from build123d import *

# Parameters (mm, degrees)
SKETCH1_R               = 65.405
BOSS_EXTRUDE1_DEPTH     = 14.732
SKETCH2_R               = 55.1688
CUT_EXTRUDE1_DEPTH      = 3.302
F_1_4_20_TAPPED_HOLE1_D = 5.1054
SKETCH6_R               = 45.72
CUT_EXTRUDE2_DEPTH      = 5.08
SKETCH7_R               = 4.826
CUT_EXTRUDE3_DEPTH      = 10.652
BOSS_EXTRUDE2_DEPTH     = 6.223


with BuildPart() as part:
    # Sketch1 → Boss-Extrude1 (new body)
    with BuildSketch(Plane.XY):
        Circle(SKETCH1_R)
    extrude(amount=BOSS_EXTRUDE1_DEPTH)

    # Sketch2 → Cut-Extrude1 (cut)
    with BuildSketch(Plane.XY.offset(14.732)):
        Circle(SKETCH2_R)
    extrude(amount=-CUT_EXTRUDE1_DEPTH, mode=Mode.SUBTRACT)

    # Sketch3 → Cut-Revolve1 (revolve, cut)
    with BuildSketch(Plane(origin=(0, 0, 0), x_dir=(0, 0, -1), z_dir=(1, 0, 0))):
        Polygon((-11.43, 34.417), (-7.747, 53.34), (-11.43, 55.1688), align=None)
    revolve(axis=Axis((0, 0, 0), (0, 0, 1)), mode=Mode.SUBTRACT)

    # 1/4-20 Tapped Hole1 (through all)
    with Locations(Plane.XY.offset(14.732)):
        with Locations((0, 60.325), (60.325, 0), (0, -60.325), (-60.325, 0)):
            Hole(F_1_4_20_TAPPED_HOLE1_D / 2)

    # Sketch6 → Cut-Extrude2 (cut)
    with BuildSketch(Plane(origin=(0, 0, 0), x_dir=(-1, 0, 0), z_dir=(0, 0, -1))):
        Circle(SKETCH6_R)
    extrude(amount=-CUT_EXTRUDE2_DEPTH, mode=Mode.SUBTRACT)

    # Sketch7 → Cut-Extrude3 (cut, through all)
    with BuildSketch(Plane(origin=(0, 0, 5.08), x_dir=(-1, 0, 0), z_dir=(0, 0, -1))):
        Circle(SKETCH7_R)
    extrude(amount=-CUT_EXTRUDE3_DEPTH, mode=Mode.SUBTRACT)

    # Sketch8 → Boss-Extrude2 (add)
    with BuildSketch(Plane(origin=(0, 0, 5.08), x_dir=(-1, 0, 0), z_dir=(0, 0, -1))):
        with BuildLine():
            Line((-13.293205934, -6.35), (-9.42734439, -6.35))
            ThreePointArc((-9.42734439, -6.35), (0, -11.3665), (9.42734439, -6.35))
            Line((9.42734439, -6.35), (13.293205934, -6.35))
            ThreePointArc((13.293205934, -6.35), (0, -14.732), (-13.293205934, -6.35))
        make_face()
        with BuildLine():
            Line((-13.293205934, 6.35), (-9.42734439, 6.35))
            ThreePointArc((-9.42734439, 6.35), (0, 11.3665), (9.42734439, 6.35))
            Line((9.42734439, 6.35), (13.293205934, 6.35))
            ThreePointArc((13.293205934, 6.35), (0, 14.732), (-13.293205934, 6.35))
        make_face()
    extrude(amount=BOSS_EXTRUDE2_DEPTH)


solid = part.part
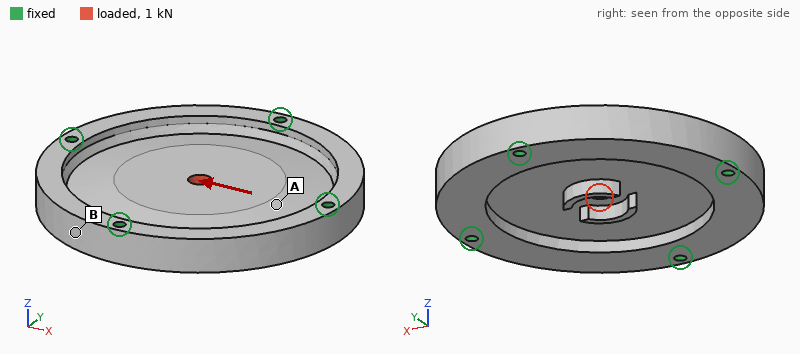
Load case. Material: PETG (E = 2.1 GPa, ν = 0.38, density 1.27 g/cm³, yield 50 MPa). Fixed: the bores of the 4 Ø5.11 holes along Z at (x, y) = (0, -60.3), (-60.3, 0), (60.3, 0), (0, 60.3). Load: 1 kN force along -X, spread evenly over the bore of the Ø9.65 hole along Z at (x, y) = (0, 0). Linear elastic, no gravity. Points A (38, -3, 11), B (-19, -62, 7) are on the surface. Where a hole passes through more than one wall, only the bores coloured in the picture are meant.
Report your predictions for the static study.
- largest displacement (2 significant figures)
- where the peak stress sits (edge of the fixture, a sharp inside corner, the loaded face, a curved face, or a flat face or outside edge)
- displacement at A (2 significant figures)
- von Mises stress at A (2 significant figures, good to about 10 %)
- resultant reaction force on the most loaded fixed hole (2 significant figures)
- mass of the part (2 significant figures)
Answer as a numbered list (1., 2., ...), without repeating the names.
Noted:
1. 74 µm
2. the loaded face
3. 34 µm
4. 1.8 MPa
5. 280 N
6. 150 g
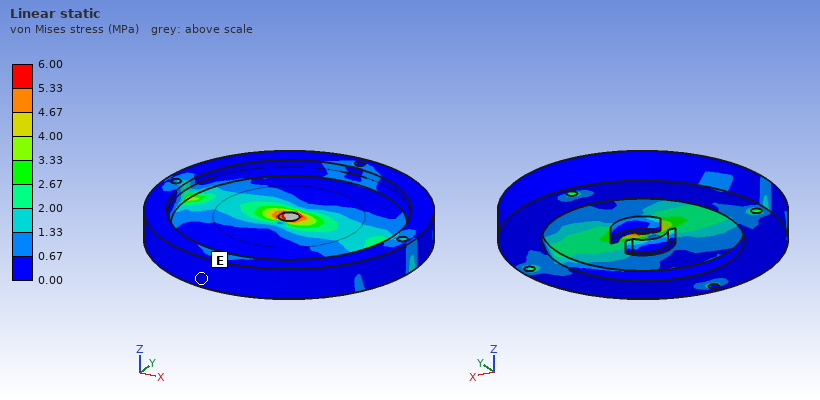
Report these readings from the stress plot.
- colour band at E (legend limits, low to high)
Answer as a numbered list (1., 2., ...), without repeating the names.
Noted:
1. 0.00 to 0.67 MPa
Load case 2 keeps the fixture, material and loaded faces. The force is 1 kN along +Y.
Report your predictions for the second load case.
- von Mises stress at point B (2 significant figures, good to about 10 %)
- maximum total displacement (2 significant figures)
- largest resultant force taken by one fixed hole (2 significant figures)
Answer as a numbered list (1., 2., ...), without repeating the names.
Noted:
1. 0.61 MPa
2. 74 µm
3. 280 N
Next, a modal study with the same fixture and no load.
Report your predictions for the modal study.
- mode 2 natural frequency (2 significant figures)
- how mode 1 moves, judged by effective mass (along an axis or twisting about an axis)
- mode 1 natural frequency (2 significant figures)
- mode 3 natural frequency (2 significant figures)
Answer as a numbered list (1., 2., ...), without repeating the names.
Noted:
1. 1700 Hz
2. along Z
3. 1100 Hz
4. 1700 Hz
